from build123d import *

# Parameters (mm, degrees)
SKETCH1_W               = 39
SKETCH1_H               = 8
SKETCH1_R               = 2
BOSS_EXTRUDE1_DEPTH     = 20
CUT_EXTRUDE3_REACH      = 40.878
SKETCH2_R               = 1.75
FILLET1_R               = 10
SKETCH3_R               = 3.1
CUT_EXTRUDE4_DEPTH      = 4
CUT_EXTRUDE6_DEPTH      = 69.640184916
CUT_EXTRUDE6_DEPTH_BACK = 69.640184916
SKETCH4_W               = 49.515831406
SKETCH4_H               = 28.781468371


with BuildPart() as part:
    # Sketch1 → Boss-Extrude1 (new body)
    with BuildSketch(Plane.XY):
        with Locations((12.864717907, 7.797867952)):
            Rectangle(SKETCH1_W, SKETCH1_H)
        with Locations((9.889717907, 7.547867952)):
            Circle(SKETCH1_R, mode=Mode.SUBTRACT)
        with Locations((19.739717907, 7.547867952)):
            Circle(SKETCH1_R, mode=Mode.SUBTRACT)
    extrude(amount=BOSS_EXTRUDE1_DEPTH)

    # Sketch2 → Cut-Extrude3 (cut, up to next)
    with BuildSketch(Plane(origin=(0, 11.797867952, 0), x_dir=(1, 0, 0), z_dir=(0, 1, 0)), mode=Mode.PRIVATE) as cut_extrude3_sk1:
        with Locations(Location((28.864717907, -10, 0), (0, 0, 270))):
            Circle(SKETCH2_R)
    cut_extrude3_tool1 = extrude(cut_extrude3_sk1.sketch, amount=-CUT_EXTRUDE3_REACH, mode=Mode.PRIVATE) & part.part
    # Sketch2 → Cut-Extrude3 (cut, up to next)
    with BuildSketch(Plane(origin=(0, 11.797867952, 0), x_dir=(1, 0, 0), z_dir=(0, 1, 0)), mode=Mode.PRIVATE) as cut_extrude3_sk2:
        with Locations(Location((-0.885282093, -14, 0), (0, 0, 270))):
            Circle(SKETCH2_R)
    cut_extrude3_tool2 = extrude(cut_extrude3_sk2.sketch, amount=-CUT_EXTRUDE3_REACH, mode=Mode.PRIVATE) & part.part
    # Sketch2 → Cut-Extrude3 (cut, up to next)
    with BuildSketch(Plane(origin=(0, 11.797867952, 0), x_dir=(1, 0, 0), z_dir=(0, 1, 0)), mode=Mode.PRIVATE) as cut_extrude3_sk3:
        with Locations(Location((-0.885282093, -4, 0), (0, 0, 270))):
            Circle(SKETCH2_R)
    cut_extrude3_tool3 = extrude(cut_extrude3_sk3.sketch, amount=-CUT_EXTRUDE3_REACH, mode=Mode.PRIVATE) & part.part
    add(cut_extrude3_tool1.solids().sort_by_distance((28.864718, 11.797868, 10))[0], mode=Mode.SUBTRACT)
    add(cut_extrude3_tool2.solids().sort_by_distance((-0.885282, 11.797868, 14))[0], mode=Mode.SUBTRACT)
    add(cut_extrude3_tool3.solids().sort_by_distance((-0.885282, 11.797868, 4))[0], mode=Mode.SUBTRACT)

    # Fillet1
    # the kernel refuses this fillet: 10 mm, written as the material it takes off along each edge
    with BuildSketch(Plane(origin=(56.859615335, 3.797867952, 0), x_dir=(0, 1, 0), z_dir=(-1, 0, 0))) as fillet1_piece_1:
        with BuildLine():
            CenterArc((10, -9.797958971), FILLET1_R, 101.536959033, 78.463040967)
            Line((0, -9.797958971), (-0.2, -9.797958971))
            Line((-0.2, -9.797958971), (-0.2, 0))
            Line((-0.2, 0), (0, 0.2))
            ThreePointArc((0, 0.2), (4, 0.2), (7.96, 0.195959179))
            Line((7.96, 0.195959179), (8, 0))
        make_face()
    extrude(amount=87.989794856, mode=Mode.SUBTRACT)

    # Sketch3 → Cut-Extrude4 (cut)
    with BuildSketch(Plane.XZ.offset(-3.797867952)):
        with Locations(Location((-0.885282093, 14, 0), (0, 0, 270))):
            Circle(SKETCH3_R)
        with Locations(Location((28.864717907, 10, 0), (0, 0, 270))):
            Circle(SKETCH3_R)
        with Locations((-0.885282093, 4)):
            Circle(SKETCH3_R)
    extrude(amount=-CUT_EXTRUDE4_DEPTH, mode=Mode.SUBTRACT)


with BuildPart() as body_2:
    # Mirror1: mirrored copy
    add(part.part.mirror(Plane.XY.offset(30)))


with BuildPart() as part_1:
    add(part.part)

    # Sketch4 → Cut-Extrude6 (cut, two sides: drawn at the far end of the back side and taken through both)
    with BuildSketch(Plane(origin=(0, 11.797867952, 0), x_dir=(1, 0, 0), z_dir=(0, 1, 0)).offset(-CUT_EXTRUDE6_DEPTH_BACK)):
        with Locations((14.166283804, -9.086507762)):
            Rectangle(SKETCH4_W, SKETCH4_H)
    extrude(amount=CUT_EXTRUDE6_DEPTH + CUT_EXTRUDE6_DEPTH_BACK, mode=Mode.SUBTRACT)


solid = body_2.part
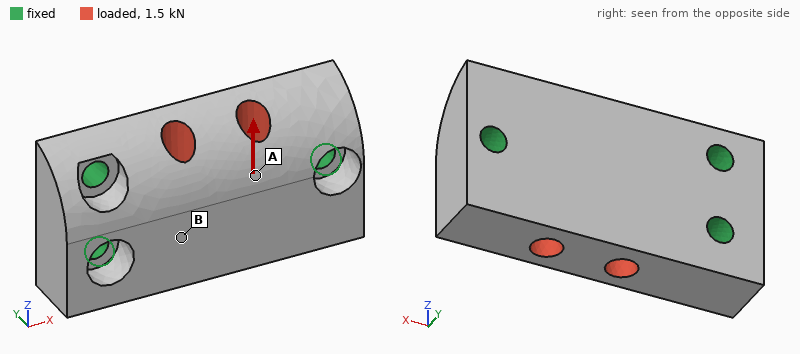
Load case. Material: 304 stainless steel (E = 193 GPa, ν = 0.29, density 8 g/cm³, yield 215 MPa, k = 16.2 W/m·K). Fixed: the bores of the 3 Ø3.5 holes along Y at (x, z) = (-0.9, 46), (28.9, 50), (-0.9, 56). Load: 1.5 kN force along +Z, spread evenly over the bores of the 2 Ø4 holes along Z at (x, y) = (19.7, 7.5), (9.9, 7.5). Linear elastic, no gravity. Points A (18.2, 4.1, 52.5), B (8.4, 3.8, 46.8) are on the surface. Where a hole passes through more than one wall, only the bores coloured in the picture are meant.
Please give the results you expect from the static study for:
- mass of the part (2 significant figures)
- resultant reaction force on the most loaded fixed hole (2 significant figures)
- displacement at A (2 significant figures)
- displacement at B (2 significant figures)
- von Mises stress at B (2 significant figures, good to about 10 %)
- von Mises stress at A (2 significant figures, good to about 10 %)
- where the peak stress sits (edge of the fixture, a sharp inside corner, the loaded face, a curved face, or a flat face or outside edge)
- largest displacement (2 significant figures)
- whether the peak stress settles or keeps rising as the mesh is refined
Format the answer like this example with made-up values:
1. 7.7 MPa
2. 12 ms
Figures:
1. 37 g
2. 650 N
3. 2.3 µm
4. 1.8 µm
5. 21 MPa
6. 9.1 MPa
7. edge of the fixture
8. 2.6 µm
9. keeps rising
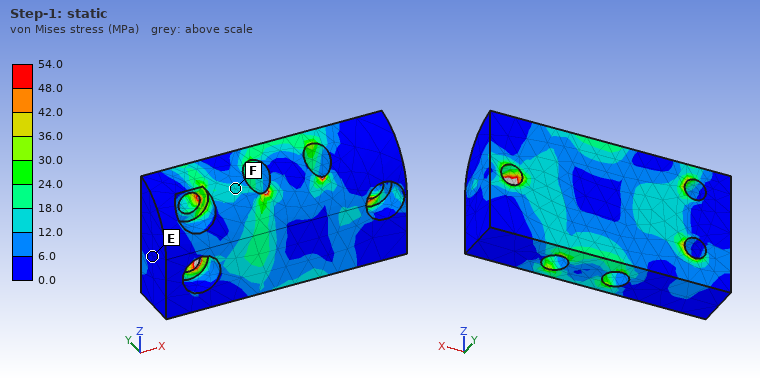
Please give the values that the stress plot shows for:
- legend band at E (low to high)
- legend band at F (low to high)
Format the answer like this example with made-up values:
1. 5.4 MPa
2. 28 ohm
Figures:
1. 0.0 to 6.0 MPa
2. 12.0 to 18.0 MPa
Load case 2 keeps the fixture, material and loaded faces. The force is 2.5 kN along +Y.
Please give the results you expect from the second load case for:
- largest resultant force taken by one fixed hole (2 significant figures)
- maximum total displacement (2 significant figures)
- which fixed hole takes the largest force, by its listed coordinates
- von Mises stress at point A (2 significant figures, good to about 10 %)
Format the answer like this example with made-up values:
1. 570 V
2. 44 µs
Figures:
1. 1.3 kN
2. 8.0 µm
3. (28.9, 50)
4. 78 MPa
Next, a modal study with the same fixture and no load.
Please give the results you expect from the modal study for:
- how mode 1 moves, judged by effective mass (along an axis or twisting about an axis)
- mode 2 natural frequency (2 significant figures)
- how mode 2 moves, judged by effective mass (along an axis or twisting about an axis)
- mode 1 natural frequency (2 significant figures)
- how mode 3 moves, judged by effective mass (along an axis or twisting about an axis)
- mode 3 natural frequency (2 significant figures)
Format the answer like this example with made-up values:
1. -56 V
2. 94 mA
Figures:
1. along Y
2. 25 kHz
3. along Y
4. 22 kHz
5. along Z
6. 35 kHz
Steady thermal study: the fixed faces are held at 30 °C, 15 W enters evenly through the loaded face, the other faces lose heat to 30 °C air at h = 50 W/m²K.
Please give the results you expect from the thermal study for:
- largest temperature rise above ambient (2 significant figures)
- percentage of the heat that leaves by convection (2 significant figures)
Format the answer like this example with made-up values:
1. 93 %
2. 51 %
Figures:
1. 48 K
2. 17 %
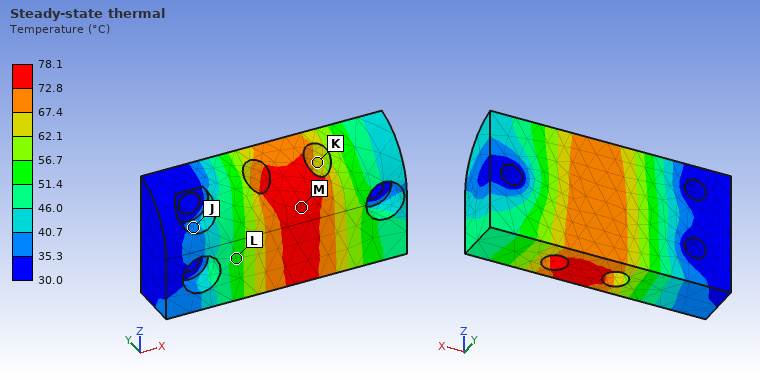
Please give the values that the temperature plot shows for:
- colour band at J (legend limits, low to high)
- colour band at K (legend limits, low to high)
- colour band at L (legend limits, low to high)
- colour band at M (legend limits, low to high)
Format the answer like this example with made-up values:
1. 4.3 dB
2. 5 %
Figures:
1. 35.3 to 40.7 °C
2. 62.1 to 67.4 °C
3. 51.4 to 56.7 °C
4. 72.8 to 78.1 °C
